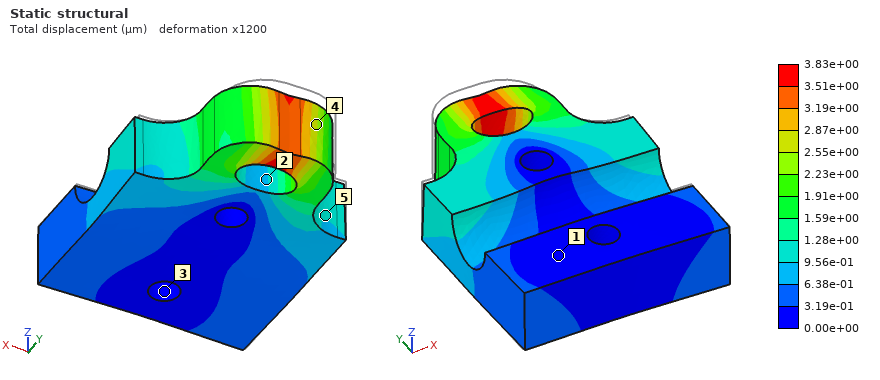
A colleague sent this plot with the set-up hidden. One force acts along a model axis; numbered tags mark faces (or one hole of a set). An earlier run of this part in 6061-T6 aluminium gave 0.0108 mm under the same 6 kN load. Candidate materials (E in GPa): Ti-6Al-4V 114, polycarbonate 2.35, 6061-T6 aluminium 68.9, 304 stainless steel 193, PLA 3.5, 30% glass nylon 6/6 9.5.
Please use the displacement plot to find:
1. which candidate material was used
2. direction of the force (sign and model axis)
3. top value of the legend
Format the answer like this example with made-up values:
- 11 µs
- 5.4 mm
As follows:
- 304 stainless steel
- -Y
- 3.83e+00 µm
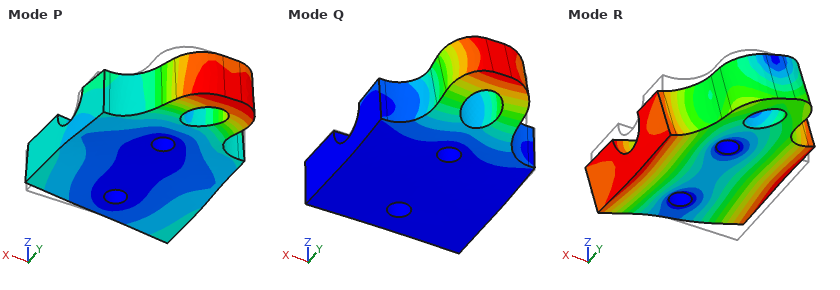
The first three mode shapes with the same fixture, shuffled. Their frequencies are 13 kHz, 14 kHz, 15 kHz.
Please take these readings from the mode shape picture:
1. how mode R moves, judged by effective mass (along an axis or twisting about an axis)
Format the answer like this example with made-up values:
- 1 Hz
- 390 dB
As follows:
- twisting about Y
